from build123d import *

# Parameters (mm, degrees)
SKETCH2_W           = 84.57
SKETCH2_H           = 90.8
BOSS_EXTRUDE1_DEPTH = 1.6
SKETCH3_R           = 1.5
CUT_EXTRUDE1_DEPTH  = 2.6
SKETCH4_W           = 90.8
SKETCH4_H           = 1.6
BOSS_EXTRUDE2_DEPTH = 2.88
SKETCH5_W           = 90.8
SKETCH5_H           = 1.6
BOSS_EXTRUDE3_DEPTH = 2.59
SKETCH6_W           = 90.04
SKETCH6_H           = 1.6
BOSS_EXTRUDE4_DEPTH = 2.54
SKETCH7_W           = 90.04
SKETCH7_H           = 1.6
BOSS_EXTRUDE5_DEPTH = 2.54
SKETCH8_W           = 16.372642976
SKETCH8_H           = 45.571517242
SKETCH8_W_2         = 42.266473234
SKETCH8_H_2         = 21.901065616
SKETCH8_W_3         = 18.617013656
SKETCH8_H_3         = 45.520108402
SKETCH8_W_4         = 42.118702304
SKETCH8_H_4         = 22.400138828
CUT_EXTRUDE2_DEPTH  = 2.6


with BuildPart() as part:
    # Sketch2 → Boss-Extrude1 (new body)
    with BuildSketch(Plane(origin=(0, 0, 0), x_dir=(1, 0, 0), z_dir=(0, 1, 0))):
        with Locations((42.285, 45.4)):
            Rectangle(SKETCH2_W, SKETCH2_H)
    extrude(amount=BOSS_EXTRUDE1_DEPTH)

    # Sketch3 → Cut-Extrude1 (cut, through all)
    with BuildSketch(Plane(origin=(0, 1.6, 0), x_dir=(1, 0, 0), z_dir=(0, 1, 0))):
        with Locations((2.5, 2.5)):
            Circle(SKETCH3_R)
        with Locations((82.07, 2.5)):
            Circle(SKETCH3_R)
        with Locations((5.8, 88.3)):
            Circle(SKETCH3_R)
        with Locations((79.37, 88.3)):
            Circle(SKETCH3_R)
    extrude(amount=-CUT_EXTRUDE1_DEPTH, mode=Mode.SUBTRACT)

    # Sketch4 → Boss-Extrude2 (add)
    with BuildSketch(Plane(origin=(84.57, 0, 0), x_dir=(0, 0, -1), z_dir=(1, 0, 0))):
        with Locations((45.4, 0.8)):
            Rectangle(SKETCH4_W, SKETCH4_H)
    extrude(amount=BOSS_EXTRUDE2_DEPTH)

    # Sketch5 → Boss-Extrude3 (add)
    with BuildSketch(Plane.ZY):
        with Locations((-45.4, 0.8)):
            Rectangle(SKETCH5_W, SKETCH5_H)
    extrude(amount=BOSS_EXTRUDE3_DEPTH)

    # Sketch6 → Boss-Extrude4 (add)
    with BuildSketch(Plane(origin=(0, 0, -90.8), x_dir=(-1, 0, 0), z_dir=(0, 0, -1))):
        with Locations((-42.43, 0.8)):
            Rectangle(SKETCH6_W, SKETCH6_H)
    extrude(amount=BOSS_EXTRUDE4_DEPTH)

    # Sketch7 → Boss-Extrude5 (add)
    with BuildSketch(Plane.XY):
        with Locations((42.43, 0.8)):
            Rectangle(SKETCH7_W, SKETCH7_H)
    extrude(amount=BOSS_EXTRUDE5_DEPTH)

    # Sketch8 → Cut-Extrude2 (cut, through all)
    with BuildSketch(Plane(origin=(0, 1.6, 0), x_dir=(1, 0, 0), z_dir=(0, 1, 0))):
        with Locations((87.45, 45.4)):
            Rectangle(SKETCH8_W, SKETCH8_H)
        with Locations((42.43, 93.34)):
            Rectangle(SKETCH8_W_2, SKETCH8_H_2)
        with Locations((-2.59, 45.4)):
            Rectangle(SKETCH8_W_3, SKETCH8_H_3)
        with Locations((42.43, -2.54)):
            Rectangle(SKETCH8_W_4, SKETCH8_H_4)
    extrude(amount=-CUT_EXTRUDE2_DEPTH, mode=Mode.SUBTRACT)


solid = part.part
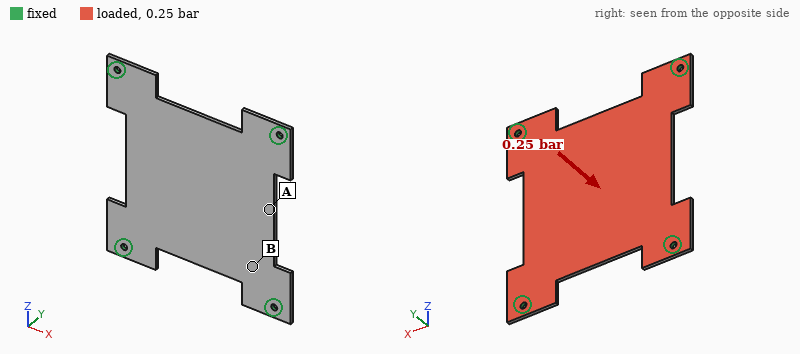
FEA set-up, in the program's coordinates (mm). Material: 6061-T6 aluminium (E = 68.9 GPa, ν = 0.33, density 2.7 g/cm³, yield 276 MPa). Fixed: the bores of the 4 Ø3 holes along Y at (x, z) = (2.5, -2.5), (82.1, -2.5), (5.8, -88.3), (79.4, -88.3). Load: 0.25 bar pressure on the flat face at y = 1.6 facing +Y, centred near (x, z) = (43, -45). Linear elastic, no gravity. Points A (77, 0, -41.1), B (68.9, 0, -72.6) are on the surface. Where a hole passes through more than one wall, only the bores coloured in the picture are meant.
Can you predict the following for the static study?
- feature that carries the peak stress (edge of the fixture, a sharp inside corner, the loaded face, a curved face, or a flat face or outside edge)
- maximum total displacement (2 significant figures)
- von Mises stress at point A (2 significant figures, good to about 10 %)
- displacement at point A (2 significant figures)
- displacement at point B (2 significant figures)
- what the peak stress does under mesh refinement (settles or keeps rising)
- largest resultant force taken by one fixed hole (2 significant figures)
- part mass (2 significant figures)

edge of the fixture
0.33 mm
26 MPa
0.24 mm
0.13 mm
keeps rising
44 N
30 g
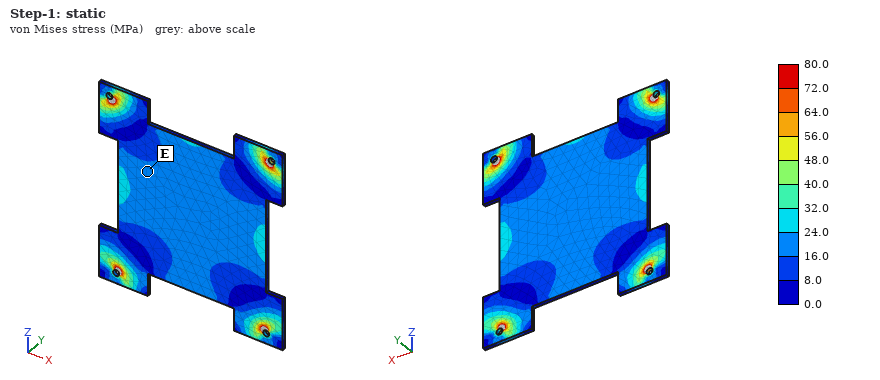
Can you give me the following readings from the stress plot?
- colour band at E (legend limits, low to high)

16.0 to 24.0 MPa
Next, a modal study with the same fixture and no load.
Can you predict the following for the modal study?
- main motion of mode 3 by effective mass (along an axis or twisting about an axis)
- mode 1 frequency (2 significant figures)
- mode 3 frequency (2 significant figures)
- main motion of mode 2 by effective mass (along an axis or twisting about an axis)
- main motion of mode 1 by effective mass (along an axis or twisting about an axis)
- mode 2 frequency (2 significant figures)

twisting about X
780 Hz
1600 Hz
twisting about Z
along Y
1400 Hz
